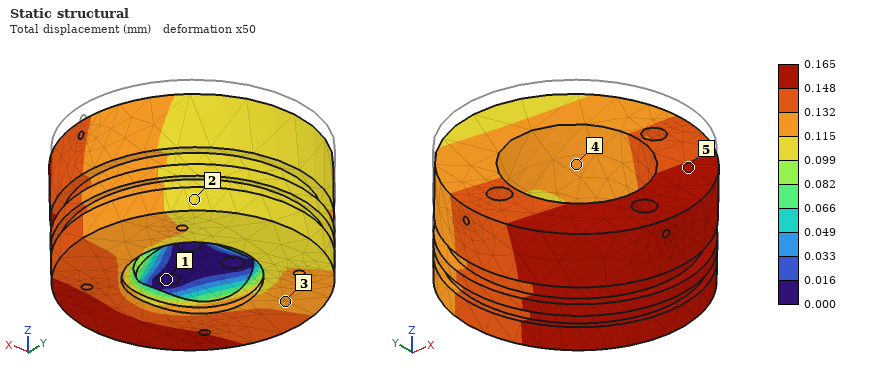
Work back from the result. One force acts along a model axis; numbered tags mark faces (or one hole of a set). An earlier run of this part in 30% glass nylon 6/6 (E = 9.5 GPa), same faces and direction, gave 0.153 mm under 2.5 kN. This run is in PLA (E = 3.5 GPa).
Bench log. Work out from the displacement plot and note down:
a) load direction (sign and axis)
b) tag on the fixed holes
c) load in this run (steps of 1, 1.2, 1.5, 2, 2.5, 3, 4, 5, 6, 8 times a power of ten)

-Z
1
1 kN
